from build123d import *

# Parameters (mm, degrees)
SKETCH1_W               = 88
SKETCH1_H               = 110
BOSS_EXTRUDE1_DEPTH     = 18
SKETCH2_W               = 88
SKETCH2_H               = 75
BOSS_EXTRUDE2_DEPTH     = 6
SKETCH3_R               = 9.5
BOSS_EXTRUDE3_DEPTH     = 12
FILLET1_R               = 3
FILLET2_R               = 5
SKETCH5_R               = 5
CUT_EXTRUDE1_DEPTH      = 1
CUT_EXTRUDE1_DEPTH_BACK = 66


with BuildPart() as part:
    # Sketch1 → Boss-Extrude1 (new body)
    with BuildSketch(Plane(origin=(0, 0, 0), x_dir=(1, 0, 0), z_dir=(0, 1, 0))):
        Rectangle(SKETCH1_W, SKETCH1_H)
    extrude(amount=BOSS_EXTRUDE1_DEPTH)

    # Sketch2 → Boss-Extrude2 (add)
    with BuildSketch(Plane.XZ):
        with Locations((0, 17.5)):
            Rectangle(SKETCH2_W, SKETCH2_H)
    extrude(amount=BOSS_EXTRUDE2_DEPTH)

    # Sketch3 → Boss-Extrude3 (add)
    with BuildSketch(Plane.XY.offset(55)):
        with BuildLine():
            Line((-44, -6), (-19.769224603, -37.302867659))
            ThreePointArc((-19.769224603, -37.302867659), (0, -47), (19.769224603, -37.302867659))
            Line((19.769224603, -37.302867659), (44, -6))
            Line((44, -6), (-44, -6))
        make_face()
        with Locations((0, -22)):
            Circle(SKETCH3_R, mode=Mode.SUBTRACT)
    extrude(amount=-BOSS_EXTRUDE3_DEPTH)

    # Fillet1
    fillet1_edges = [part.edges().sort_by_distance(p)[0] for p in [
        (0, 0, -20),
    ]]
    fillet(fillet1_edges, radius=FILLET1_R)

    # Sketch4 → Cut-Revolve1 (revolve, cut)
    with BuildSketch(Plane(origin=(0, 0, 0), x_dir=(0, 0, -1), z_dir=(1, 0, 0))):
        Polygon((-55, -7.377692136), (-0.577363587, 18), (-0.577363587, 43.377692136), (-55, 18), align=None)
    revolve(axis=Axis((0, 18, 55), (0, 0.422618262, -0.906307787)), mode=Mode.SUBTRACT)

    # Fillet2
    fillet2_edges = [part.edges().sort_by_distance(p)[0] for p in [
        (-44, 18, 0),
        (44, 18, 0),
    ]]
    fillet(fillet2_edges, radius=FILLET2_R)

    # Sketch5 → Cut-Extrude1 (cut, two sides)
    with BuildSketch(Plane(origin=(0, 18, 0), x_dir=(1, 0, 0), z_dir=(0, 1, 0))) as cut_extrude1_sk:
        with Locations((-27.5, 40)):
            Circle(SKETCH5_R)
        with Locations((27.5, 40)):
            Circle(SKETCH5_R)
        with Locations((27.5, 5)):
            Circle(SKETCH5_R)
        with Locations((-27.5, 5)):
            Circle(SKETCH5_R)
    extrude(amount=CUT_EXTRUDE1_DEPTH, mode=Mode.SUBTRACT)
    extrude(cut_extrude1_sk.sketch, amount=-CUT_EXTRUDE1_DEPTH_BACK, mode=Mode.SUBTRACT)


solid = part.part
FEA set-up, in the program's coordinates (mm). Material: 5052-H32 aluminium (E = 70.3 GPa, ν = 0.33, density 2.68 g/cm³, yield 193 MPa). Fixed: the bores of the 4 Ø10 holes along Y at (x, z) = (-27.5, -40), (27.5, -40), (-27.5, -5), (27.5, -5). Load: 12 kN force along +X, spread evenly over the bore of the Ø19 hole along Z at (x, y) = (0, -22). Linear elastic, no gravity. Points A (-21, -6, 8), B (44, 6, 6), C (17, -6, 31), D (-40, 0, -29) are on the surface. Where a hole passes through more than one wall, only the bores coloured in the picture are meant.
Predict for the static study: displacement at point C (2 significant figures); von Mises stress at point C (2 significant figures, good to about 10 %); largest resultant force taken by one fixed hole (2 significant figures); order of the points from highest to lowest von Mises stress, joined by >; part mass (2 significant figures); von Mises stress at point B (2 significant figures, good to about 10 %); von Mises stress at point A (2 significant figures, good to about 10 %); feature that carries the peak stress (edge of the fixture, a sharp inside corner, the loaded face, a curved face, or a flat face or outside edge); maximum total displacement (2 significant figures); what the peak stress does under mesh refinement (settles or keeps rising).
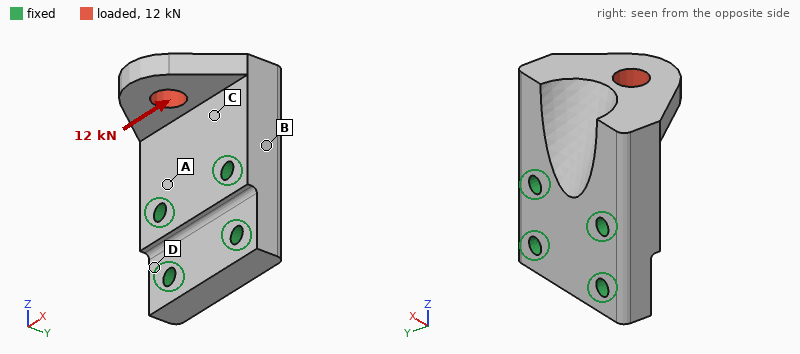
0.028 mm
45 MPa
12 kN
C > A > B > D
560 g
26 MPa
33 MPa
edge of the fixture
0.11 mm
keeps rising
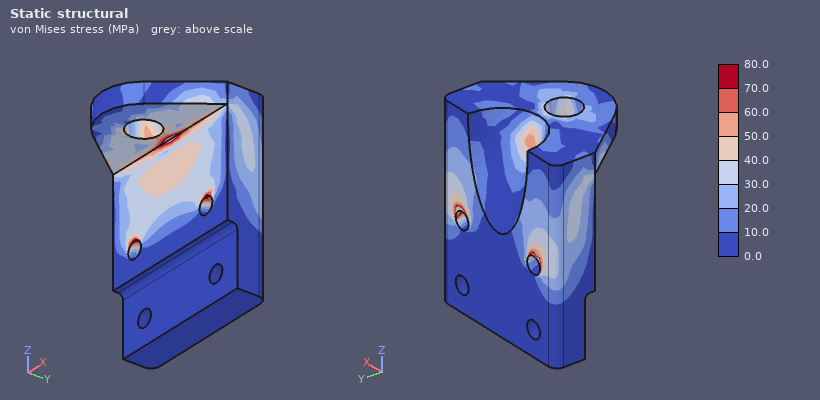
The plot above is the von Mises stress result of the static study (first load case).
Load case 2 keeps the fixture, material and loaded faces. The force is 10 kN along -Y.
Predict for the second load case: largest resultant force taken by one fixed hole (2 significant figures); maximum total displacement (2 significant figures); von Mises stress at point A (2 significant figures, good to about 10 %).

6.6 kN
0.20 mm
56 MPa
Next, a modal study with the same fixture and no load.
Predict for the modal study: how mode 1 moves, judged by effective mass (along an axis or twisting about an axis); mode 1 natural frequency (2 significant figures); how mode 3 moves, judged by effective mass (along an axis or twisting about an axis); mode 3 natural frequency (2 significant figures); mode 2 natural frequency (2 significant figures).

along Y
3400 Hz
along Y
5900 Hz
5200 Hz
